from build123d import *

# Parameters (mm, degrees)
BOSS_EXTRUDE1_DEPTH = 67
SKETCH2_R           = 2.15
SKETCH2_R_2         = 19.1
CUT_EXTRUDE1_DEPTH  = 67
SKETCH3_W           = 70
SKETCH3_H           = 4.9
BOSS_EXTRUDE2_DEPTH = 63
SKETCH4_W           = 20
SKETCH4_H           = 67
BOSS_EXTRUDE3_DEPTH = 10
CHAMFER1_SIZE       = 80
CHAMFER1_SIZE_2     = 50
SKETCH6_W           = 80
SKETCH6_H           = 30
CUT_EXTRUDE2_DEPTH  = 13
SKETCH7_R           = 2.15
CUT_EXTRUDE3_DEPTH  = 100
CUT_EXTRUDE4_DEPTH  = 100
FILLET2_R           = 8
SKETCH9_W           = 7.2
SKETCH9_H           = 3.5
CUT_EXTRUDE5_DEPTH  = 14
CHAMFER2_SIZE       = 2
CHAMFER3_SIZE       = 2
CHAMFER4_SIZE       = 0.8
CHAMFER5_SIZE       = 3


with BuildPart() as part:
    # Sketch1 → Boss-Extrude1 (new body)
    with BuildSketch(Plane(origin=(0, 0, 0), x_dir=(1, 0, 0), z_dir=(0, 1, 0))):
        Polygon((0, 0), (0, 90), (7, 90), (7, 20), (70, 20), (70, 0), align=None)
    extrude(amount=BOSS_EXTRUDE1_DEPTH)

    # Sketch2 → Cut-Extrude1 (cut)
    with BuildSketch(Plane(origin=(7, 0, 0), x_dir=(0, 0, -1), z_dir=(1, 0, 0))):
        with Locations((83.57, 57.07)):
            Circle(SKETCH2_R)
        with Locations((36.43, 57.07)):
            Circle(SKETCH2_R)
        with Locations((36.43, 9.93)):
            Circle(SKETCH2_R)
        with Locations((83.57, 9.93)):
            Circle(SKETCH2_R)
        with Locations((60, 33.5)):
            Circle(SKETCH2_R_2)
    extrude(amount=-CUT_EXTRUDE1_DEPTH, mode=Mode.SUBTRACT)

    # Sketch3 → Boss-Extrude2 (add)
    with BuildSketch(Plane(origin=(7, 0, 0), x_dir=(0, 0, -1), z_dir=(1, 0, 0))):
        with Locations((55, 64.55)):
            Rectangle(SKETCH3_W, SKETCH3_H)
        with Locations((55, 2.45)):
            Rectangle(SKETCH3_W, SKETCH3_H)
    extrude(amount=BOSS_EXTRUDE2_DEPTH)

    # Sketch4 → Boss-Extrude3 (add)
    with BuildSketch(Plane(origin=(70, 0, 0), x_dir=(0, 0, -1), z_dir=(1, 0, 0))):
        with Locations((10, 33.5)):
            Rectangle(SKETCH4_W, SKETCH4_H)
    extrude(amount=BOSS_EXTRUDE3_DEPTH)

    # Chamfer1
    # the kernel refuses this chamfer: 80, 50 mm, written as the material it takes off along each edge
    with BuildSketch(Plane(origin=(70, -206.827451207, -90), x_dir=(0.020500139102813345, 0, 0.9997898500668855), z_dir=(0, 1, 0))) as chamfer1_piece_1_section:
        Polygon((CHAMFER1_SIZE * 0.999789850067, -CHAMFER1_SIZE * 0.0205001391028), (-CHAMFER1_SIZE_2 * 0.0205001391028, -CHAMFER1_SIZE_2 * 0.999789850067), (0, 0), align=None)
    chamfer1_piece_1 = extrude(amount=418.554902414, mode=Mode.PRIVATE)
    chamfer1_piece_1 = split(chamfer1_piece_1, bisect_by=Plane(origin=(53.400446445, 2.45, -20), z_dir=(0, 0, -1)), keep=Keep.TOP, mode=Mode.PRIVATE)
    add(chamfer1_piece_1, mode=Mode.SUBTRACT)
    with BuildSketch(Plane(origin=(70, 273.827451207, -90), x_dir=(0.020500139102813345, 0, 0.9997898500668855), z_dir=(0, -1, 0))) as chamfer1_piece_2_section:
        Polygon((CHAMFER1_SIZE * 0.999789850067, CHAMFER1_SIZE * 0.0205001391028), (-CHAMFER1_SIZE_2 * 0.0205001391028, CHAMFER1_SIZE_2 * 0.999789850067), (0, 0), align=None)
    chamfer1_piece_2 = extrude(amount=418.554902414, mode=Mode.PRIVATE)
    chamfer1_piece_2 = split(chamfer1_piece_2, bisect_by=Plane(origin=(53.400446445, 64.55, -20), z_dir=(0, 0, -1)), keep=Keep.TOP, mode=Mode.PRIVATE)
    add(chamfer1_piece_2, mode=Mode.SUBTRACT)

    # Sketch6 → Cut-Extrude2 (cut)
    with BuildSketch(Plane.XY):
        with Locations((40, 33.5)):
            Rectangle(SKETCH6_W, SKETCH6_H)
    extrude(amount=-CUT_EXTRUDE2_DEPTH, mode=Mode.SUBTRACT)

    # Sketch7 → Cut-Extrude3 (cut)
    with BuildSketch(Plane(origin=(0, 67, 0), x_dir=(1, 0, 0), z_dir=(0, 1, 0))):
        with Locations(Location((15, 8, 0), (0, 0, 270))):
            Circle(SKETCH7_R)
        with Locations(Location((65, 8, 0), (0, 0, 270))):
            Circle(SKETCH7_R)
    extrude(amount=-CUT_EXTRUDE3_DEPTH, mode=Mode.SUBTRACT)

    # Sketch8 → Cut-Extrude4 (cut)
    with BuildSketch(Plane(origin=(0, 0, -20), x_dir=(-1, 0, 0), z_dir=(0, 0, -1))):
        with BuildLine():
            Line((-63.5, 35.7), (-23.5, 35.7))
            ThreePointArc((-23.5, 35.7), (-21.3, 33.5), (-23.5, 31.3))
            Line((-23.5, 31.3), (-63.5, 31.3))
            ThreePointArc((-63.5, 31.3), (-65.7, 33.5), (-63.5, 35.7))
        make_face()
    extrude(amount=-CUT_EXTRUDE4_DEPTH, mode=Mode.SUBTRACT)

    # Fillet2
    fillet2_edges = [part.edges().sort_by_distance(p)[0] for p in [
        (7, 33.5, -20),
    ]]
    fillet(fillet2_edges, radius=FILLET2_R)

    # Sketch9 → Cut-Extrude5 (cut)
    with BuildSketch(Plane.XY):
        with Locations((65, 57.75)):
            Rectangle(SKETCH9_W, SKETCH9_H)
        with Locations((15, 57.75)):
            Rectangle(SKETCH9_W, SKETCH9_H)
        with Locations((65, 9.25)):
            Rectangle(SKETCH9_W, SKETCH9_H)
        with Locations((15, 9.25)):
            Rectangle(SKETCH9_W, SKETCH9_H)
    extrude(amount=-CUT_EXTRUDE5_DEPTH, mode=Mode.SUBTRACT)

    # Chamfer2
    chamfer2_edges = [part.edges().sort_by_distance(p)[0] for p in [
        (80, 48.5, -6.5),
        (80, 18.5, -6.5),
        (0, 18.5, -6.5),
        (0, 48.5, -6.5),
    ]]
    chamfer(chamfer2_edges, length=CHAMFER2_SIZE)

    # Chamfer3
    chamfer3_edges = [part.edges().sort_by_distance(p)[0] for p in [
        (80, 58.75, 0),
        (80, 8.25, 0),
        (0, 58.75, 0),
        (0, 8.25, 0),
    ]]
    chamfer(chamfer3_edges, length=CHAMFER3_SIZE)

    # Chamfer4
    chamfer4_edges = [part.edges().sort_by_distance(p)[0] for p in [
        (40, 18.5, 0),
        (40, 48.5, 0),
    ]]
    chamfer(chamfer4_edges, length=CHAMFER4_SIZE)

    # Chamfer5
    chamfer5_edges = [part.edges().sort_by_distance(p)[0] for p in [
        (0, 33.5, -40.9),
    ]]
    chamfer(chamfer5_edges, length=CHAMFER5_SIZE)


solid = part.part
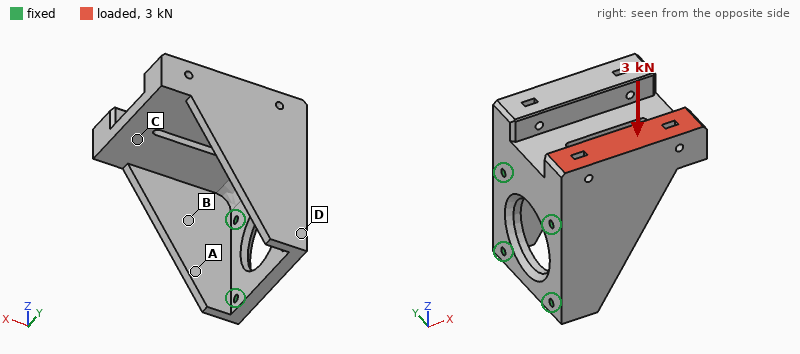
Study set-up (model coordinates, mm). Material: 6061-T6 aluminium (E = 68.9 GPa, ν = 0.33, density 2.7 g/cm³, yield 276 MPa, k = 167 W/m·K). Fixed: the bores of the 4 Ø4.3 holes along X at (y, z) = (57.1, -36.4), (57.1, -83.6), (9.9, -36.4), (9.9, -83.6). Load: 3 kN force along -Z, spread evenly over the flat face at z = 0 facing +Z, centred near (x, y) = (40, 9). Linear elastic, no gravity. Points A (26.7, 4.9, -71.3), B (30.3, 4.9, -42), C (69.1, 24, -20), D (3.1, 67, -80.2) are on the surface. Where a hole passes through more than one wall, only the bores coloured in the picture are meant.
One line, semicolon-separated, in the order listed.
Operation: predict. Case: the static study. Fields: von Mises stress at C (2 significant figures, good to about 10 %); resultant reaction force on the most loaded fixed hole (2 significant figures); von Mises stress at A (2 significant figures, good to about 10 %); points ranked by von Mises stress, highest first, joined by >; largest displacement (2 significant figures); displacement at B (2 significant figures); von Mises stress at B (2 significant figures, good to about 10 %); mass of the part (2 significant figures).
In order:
21 MPa; 2.3 kN; 27 MPa; A > C > B > D; 0.10 mm; 0.026 mm; 16 MPa; 330 g
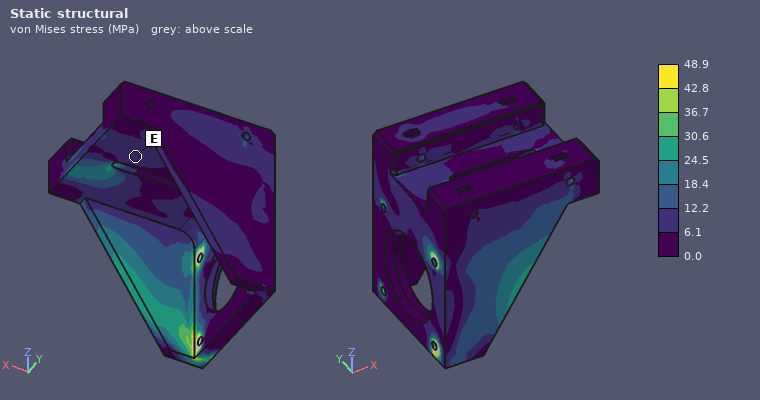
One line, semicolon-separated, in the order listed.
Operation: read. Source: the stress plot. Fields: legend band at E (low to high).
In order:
6.1 to 12.2 MPa
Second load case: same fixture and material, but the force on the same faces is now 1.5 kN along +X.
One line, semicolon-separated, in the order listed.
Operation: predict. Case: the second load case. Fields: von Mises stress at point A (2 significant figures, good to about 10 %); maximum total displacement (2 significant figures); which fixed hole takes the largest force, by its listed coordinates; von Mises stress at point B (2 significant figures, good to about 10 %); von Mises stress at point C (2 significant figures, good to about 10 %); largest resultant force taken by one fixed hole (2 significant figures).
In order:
13 MPa; 67 µm; (9.9, -36.4); 6.1 MPa; 9.7 MPa; 2.3 kN
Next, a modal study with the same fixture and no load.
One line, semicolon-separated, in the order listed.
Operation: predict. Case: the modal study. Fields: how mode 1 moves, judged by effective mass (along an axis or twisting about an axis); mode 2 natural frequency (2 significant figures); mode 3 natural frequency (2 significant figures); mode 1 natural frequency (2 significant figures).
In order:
along Y; 2400 Hz; 4700 Hz; 2200 Hz
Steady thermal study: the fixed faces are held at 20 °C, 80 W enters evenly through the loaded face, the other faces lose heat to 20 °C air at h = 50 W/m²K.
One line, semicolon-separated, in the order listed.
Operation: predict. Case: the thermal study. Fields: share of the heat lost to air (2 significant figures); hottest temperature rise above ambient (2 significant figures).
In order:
27 %; 36 K
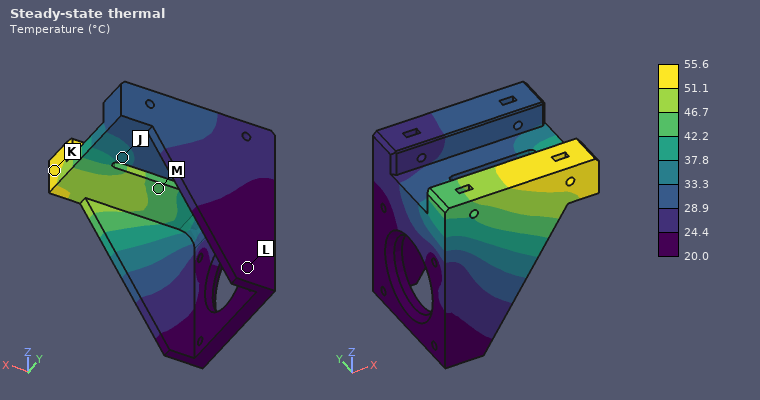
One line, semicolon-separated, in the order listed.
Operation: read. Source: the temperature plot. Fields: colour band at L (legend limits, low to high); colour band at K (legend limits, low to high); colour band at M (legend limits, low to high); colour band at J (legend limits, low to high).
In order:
20.0 to 24.4 °C; 51.1 to 55.6 °C; 42.2 to 46.7 °C; 33.3 to 37.8 °C
